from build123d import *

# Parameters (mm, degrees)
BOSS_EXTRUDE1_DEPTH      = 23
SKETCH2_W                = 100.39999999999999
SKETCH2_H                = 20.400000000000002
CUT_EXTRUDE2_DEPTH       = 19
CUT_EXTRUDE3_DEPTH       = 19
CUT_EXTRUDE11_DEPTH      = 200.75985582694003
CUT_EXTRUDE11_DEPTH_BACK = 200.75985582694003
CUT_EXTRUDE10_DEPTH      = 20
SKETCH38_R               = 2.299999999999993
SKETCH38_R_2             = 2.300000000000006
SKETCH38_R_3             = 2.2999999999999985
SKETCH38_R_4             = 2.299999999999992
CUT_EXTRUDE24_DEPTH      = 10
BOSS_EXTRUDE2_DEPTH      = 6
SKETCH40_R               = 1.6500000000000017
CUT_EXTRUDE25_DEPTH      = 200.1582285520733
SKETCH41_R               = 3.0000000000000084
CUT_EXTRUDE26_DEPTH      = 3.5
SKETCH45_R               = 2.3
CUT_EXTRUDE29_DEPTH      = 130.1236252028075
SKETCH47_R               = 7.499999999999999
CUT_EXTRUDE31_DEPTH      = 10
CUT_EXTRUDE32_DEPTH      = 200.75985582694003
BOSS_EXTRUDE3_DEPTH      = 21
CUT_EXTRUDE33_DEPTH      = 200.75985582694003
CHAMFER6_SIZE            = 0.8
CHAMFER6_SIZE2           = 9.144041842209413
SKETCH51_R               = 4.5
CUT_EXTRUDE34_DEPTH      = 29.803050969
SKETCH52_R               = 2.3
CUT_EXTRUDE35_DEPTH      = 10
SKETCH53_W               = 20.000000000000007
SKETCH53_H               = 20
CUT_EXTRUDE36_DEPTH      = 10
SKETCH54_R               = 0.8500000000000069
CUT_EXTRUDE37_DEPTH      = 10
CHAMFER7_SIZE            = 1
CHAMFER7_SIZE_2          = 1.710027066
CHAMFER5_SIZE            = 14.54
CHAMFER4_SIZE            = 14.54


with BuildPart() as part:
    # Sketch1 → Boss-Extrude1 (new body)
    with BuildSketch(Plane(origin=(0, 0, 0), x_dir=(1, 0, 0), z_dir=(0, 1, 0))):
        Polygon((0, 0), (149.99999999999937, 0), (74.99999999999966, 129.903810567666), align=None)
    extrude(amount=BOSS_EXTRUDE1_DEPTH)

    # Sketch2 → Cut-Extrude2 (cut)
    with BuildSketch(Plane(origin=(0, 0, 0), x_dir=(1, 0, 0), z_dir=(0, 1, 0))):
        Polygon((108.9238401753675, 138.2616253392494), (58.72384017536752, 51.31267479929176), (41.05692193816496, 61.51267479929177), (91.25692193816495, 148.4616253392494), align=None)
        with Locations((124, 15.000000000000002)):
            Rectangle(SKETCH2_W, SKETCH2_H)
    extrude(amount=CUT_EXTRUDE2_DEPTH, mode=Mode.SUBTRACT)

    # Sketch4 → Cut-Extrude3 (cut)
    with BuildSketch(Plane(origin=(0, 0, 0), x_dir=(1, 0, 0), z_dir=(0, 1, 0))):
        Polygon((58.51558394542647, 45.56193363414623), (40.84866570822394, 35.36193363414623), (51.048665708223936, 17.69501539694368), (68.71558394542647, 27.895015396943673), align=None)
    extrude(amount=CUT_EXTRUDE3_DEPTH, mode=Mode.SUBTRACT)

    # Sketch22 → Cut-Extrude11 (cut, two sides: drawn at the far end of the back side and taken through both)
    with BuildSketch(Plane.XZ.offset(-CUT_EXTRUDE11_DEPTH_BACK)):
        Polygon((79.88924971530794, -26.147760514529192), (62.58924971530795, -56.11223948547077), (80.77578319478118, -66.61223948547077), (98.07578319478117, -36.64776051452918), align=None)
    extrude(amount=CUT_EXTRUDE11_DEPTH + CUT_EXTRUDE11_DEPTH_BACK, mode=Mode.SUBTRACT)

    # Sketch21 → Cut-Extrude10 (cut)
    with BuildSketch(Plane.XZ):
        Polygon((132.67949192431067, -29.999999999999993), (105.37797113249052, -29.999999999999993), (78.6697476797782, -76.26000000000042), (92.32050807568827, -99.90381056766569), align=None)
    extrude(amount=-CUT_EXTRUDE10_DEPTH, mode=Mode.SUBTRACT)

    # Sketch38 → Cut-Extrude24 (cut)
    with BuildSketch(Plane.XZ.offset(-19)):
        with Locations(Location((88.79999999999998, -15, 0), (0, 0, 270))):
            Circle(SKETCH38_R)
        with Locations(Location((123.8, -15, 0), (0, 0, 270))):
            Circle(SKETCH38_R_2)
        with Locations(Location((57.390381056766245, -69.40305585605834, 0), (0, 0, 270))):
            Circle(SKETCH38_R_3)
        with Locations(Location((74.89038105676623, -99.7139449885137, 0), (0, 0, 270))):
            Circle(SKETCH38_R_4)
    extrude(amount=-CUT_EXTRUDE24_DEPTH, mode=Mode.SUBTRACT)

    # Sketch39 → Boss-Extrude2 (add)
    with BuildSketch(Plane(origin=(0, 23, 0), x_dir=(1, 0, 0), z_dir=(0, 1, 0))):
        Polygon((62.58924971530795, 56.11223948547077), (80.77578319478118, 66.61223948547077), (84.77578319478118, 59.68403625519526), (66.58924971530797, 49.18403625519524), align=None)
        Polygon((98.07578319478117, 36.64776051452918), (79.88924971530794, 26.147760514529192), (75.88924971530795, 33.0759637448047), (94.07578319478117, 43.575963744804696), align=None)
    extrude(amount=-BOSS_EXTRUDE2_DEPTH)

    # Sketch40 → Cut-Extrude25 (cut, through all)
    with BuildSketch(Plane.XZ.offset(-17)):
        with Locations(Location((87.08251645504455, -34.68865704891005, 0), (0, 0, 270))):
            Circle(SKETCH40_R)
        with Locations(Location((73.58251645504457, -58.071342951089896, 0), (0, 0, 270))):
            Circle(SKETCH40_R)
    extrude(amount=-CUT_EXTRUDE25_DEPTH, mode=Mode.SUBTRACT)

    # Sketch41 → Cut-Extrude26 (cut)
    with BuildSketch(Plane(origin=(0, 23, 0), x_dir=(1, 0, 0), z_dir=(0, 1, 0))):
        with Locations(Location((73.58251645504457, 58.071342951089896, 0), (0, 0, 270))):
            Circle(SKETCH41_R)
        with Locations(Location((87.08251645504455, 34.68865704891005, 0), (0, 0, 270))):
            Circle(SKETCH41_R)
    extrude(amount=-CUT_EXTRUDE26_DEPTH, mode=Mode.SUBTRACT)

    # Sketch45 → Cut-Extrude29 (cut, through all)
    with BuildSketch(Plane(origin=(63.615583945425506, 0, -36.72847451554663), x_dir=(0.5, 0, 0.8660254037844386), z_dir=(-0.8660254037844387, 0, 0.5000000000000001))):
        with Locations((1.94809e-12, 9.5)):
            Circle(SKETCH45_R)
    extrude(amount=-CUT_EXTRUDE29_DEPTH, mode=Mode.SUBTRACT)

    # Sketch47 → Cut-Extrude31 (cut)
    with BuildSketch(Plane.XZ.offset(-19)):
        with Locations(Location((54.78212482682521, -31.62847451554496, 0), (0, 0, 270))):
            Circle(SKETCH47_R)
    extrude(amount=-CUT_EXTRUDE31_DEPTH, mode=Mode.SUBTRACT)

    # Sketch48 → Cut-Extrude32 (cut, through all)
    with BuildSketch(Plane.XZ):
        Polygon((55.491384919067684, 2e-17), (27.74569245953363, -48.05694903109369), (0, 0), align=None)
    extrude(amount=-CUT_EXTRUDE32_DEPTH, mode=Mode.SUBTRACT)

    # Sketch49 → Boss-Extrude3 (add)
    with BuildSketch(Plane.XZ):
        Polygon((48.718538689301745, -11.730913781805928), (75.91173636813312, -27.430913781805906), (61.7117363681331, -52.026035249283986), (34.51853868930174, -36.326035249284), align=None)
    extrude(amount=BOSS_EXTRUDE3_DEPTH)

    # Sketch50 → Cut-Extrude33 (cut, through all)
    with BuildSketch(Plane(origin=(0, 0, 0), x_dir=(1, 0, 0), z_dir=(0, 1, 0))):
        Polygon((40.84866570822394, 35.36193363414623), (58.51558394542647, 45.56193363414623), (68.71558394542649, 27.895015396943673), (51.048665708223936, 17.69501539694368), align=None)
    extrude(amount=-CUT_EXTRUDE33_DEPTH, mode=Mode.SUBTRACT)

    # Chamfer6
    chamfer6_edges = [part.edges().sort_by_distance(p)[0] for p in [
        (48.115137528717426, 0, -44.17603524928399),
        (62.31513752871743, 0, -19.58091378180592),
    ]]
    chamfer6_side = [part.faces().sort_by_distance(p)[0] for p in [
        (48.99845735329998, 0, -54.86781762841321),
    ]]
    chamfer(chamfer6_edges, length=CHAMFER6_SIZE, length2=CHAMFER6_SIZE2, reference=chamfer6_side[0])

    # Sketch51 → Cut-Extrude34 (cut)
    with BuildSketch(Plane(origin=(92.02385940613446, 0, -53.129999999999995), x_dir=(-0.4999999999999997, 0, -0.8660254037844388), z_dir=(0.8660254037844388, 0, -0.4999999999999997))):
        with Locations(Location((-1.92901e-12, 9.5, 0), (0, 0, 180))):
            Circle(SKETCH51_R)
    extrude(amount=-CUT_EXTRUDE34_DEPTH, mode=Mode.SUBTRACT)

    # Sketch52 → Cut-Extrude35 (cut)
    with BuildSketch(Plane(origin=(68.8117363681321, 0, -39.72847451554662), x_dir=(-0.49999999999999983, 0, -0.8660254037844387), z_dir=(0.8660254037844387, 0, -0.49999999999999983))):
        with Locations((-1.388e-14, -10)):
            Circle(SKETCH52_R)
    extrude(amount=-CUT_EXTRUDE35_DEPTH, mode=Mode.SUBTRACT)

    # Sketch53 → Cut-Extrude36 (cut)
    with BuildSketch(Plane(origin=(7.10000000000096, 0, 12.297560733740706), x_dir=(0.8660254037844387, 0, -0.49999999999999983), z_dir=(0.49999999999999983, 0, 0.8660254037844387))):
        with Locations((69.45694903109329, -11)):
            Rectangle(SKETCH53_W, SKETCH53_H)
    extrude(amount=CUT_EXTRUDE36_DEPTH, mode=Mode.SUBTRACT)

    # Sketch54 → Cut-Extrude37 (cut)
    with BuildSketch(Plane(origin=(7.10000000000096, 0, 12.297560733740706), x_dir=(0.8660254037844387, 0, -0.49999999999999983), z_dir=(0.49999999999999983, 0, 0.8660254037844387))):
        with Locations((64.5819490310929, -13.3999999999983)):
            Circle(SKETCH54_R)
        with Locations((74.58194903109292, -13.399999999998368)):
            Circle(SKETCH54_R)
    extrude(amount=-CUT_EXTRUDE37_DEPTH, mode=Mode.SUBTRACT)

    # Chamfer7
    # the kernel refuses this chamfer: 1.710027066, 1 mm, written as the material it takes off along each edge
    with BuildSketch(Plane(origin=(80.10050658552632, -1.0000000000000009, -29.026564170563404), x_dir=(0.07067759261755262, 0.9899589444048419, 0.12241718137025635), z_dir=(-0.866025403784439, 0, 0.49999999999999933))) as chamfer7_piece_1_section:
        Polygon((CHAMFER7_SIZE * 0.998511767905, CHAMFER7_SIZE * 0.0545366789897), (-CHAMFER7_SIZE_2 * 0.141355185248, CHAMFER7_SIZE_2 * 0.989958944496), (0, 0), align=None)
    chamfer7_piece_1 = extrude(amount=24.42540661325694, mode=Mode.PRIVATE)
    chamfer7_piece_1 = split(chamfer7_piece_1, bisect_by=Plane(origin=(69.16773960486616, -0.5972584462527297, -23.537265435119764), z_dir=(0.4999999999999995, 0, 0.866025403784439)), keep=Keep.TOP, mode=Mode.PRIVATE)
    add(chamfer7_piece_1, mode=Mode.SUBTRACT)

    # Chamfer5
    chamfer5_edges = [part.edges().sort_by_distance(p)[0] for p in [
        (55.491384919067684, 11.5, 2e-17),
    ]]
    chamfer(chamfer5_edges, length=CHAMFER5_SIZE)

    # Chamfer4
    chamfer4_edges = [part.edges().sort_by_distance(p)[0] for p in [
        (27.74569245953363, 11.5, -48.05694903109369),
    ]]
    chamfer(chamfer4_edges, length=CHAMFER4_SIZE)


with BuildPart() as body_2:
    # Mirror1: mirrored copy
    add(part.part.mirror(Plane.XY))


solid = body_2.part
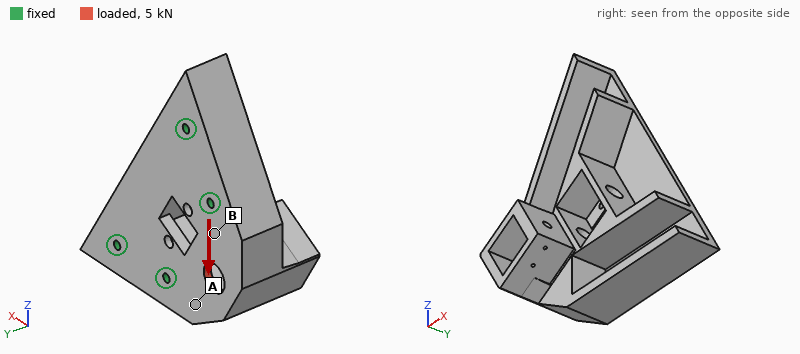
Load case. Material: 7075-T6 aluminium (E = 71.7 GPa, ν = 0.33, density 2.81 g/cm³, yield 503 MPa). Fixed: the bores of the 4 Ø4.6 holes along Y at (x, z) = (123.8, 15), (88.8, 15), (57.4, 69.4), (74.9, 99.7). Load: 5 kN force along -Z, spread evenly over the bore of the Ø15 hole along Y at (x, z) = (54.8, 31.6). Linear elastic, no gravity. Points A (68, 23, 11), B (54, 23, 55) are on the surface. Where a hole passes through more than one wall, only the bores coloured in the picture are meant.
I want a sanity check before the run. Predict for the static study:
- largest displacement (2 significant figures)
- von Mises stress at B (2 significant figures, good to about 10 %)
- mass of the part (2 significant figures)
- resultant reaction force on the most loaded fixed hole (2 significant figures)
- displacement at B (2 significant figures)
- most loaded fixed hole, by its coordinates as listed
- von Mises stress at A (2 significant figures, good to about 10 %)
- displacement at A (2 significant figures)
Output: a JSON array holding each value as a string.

["24 µm", "30 MPa", "250 g", "2.8 kN", "7.9 µm", "(57.4, 69.4)", "8.6 MPa", "14 µm"]
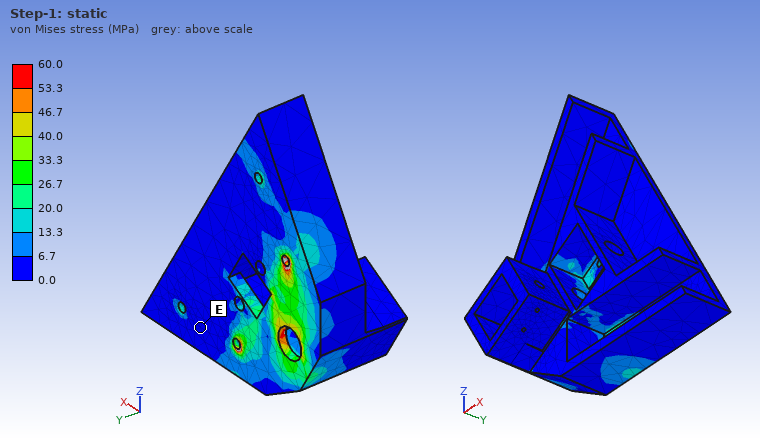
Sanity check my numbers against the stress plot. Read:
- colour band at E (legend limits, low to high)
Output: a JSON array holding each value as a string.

["0.0 to 6.7 MPa"]
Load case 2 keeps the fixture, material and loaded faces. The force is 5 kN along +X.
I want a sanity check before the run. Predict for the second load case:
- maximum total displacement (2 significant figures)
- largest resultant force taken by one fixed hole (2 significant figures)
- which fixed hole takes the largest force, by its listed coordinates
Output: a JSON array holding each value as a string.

["24 µm", "2.6 kN", "(88.8, 15)"]
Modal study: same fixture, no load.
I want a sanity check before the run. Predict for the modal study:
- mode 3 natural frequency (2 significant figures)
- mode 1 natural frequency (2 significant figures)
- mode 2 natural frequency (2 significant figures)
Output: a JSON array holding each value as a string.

["4000 Hz", "2500 Hz", "3900 Hz"]
